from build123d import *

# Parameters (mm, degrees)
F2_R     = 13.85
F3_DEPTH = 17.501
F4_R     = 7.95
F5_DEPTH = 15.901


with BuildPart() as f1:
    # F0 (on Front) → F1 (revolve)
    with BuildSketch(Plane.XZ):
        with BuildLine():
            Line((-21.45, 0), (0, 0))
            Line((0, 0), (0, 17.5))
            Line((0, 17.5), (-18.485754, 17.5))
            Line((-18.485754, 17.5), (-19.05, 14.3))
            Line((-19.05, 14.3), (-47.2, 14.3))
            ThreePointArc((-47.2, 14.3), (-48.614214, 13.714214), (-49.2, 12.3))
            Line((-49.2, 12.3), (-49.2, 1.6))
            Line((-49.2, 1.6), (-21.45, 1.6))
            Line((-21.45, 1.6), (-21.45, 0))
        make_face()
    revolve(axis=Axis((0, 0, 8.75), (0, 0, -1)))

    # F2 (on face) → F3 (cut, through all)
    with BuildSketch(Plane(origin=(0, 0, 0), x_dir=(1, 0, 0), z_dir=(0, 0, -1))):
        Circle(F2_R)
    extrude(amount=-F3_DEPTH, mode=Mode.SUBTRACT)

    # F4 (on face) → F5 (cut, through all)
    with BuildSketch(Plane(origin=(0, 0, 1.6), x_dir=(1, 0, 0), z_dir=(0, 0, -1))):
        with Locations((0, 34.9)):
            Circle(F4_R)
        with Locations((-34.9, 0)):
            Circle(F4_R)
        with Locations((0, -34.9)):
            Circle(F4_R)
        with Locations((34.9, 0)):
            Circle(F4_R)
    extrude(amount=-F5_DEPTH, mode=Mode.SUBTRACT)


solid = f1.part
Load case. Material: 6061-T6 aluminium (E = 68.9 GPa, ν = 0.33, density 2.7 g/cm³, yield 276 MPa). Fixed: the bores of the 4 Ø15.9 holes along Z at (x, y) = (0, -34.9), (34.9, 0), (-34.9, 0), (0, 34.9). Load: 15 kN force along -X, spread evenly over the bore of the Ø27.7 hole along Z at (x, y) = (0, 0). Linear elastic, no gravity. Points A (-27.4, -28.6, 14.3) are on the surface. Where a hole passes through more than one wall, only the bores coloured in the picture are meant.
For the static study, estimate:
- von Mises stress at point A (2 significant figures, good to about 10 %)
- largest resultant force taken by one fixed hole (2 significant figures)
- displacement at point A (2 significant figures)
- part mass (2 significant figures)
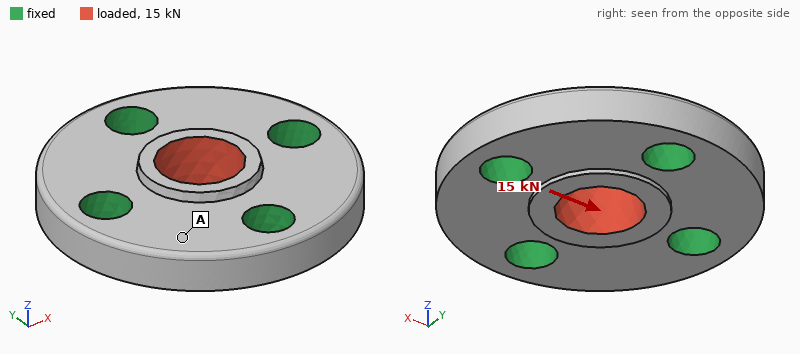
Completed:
2.6 MPa
4.9 kN
1.6 µm
220 g
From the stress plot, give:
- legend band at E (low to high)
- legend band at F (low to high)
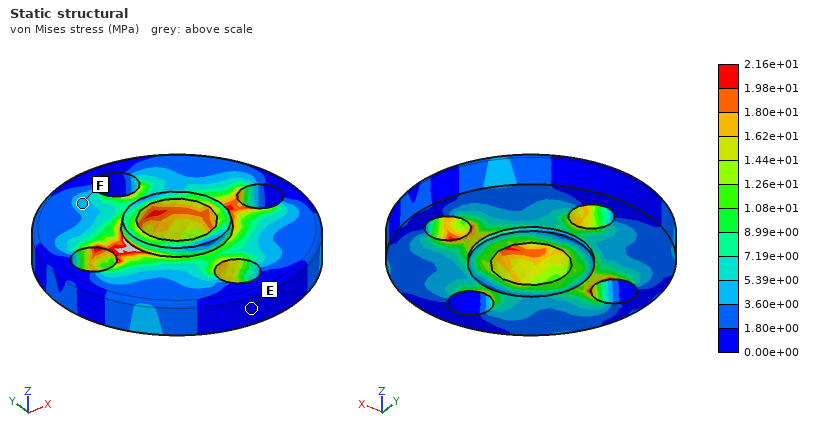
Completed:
0.00e+00 to 1.80e+00 MPa
3.60e+00 to 5.39e+00 MPa
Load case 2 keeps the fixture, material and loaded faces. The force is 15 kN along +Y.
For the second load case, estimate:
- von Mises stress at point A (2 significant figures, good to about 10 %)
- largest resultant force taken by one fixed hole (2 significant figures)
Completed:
2.6 MPa
4.9 kN
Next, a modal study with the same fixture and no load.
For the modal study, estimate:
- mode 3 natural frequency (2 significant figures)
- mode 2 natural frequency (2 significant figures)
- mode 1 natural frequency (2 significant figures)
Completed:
19 kHz
19 kHz
19 kHz
